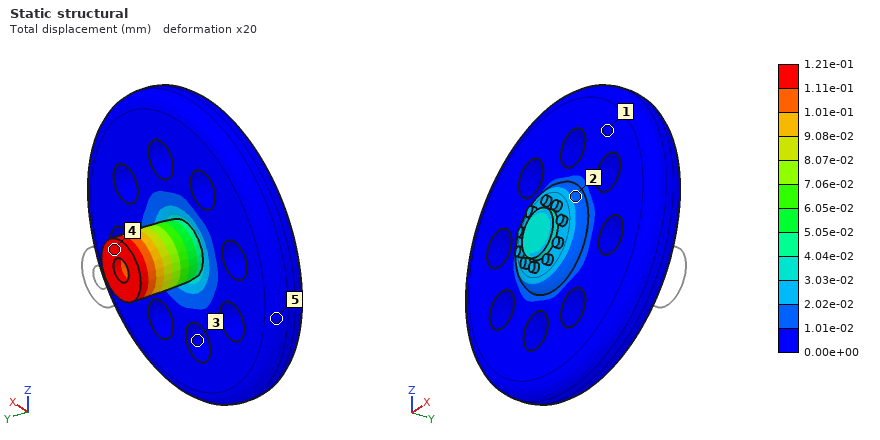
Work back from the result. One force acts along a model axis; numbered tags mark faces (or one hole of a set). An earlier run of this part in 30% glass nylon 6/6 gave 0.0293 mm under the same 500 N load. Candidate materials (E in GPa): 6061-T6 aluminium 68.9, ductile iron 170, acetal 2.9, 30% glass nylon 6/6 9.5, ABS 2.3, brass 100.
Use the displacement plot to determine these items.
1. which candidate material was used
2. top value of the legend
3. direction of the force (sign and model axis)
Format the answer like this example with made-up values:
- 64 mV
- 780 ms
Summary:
- ABS
- 1.21e-01 mm
- -Y
